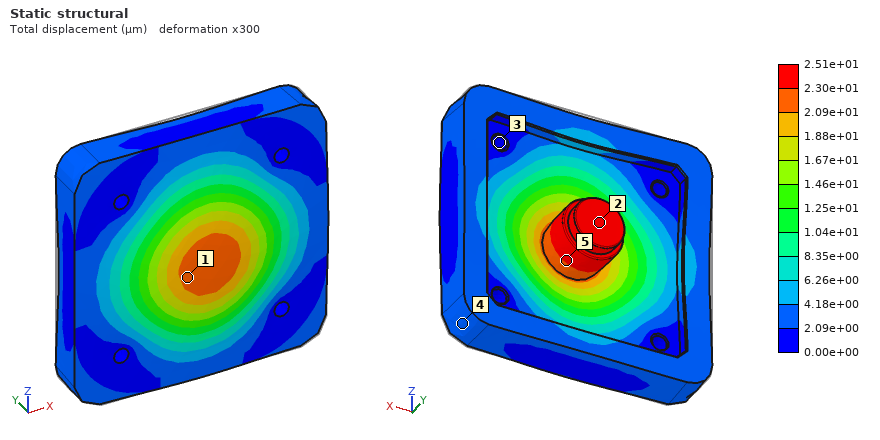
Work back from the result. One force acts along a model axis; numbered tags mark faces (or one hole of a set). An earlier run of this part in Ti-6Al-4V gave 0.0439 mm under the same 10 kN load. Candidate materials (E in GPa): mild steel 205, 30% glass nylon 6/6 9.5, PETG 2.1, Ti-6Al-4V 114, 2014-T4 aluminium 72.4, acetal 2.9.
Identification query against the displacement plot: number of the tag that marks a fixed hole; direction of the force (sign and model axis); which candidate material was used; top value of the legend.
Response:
3
-Y
mild steel
2.51e+01 µm
